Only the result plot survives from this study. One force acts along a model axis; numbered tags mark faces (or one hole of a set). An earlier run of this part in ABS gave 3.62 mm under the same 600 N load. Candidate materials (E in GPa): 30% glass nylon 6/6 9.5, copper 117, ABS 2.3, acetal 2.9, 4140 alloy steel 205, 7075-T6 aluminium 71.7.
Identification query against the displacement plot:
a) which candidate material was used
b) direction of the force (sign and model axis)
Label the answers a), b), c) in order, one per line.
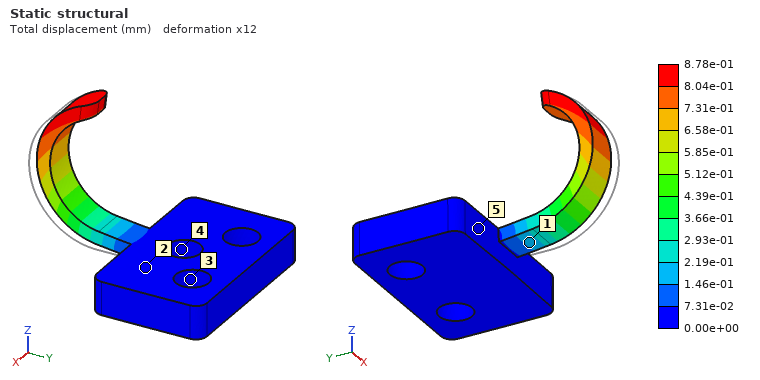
a) 30% glass nylon 6/6
b) +Z
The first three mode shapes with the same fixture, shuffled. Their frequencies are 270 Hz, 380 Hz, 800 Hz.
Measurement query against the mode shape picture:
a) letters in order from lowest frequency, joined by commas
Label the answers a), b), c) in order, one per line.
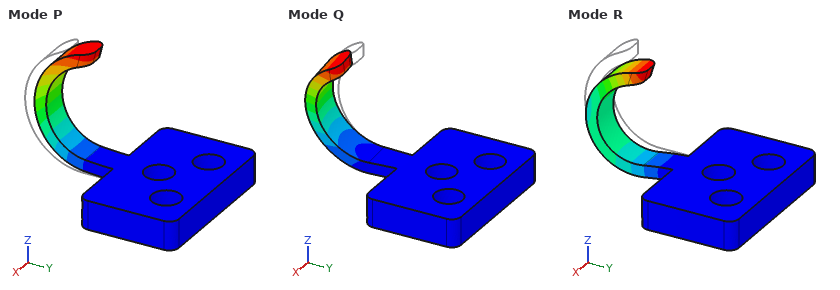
a) P, Q, R
